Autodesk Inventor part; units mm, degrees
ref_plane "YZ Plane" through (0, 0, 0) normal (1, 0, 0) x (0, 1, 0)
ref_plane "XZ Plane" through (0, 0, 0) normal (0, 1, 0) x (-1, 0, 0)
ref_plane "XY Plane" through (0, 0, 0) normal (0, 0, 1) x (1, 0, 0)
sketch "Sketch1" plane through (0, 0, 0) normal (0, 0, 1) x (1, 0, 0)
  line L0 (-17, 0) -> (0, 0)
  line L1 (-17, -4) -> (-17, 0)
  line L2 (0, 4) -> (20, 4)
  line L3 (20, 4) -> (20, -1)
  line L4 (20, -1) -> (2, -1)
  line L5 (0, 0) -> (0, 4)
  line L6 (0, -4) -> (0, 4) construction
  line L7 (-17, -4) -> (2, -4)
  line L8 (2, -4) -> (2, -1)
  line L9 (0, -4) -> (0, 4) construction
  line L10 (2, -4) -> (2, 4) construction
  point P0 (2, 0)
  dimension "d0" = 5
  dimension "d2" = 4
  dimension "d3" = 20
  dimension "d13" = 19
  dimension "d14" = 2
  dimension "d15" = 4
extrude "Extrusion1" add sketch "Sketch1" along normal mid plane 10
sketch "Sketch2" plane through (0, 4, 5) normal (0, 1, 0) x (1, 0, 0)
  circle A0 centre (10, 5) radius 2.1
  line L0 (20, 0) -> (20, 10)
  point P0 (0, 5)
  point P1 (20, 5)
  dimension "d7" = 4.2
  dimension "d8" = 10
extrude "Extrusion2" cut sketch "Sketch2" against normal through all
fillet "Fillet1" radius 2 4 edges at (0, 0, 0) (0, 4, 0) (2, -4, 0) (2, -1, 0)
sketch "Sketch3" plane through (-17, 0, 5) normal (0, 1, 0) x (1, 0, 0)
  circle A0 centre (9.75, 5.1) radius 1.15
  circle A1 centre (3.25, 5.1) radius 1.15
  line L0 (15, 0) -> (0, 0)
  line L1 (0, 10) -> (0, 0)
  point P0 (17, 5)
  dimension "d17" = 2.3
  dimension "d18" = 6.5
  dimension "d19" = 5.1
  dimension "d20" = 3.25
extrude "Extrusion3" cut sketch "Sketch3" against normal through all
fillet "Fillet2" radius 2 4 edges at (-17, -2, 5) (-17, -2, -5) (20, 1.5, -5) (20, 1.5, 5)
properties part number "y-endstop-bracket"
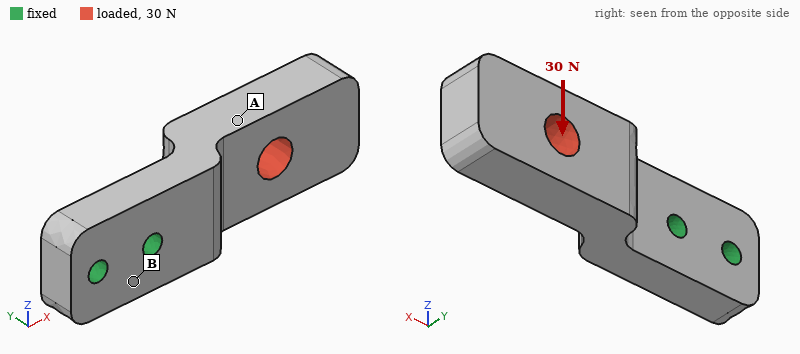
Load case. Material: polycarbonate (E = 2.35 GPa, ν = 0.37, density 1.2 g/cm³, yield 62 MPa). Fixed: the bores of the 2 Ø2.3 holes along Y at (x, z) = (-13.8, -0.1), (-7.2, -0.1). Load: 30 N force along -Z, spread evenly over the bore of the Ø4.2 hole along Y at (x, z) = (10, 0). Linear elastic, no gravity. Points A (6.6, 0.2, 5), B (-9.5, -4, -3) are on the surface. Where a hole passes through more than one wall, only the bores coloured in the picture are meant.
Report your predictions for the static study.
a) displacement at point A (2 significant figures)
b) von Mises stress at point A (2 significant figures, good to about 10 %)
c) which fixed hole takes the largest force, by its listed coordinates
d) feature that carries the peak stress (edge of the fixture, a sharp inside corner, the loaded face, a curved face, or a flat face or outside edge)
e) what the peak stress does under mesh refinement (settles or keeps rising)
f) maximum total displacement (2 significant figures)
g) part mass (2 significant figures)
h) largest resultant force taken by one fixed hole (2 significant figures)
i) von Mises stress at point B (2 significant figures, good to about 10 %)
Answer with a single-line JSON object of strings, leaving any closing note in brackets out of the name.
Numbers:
{"displacement at point A": "0.12 mm", "von Mises stress at point A": "2.1 MPa", "which fixed hole takes the largest force, by its listed coordinates": "(-7.2, -0.1)", "feature that carries the peak stress": "edge of the fixture", "what the peak stress does under mesh refinement": "keeps rising", "maximum total displacement": "0.25 mm", "part mass": "1.9 g", "largest resultant force taken by one fixed hole": "77 N", "von Mises stress at point B": "4.6 MPa"}
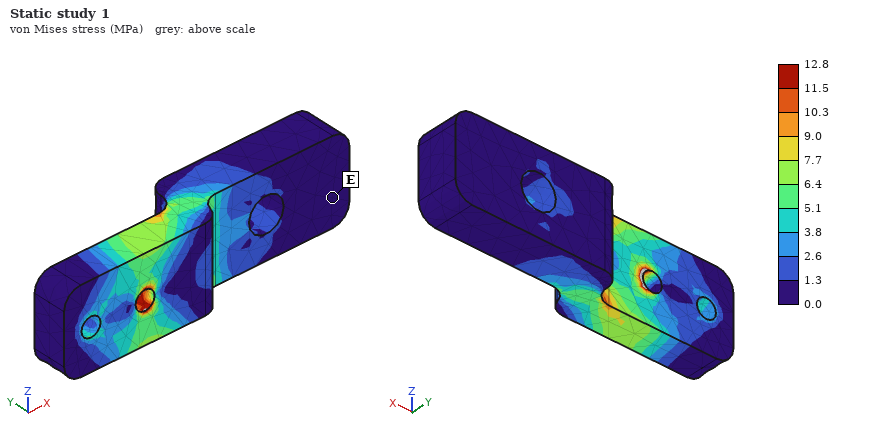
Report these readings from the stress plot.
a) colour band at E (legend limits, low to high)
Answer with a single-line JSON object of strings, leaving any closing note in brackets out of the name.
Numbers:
{"colour band at E": "0.0 to 1.3 MPa"}
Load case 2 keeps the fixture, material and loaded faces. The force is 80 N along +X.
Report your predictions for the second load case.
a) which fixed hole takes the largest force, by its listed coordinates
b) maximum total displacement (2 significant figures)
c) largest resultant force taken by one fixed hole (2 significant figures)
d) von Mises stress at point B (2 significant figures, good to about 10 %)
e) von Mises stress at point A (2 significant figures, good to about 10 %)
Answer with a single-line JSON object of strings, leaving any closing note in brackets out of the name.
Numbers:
{"which fixed hole takes the largest force, by its listed coordinates": "(-7.2, -0.1)", "maximum total displacement": "0.46 mm", "largest resultant force taken by one fixed hole": "67 N", "von Mises stress at point B": "1.6 MPa", "von Mises stress at point A": "1.5 MPa"}
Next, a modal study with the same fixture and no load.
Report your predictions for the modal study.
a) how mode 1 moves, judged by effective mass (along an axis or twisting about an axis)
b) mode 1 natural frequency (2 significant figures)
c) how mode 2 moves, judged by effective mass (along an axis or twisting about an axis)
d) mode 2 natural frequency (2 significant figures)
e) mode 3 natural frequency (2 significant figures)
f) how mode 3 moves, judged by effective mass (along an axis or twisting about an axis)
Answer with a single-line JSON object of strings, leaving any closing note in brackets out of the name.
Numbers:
{"how mode 1 moves, judged by effective mass": "along Y", "mode 1 natural frequency": "1100 Hz", "how mode 2 moves, judged by effective mass": "along Z", "mode 2 natural frequency": "1900 Hz", "mode 3 natural frequency": "4600 Hz", "how mode 3 moves, judged by effective mass": "twisting about X"}
